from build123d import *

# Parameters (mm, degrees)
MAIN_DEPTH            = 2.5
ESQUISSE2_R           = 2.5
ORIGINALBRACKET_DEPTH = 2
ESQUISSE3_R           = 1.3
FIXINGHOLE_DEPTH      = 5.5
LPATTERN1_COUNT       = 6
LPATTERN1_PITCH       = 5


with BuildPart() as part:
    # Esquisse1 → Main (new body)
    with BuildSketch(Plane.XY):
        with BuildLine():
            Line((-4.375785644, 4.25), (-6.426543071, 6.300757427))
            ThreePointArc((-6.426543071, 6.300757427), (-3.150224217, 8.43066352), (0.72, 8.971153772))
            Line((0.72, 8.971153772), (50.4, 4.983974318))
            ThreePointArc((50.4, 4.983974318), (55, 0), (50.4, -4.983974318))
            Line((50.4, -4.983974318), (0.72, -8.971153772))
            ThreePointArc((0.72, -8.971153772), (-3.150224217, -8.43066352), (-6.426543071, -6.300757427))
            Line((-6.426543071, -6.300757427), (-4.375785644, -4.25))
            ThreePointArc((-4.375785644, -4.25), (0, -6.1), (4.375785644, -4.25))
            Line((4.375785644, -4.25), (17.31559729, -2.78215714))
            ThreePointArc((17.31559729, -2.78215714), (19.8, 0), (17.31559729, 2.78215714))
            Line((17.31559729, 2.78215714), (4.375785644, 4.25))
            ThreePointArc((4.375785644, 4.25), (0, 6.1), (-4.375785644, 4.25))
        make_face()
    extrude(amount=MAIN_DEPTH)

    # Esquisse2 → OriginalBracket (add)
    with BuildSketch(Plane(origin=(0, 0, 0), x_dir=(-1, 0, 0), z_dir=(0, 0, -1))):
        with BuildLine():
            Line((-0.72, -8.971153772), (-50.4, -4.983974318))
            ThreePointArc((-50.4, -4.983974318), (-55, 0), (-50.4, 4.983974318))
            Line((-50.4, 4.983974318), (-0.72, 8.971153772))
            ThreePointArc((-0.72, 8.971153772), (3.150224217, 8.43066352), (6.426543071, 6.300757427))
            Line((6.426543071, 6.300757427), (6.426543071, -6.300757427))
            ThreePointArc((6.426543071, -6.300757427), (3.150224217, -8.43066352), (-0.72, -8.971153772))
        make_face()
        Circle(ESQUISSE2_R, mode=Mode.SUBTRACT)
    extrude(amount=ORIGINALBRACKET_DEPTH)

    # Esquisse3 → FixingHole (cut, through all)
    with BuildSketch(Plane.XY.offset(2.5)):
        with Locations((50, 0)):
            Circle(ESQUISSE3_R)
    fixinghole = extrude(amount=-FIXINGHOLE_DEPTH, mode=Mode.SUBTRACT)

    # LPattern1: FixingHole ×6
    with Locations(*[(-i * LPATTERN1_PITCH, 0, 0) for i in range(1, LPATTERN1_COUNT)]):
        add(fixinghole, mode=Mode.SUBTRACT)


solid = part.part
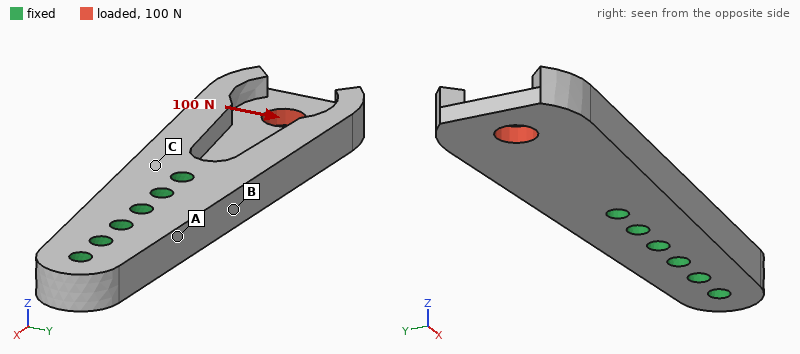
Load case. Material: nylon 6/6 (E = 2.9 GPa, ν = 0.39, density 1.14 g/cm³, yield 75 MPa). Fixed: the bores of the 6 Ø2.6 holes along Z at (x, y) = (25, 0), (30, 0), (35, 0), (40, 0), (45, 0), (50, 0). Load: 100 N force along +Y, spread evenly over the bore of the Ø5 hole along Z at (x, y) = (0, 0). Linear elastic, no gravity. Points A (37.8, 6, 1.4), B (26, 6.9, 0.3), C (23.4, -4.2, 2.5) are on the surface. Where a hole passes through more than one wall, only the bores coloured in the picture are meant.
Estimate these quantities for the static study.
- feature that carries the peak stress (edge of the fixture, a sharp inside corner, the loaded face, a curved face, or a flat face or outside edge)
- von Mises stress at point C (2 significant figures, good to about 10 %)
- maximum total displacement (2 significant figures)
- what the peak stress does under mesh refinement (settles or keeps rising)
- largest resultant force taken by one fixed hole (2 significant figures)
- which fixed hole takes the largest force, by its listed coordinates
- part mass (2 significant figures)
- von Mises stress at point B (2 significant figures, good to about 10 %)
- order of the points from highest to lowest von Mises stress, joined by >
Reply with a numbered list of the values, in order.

1. edge of the fixture
2. 8.0 MPa
3. 0.51 mm
4. keeps rising
5. 290 N
6. (25, 0)
7. 3.5 g
8. 16 MPa
9. B > C > A
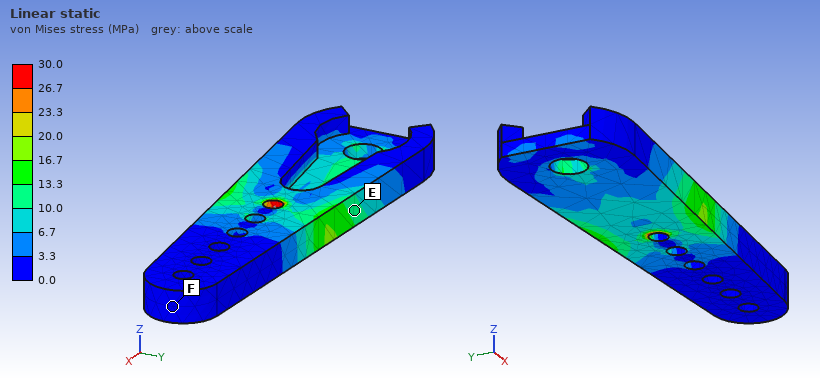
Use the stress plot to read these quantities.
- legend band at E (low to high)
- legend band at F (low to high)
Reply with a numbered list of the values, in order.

1. 10.0 to 13.3 MPa
2. 0.0 to 3.3 MPa
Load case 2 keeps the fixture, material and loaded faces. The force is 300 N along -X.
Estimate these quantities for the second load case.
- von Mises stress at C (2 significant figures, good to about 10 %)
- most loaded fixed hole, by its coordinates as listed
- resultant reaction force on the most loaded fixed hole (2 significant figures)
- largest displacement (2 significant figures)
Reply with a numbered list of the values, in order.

1. 2.4 MPa
2. (25, 0)
3. 200 N
4. 0.52 mm
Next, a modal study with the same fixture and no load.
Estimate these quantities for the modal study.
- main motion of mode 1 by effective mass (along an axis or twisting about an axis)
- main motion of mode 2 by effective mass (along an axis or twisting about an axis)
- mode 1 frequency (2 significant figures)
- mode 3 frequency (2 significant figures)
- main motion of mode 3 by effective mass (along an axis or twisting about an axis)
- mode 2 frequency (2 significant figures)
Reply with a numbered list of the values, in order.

1. along Z
2. along Y
3. 1300 Hz
4. 3000 Hz
5. along Y
6. 2500 Hz
